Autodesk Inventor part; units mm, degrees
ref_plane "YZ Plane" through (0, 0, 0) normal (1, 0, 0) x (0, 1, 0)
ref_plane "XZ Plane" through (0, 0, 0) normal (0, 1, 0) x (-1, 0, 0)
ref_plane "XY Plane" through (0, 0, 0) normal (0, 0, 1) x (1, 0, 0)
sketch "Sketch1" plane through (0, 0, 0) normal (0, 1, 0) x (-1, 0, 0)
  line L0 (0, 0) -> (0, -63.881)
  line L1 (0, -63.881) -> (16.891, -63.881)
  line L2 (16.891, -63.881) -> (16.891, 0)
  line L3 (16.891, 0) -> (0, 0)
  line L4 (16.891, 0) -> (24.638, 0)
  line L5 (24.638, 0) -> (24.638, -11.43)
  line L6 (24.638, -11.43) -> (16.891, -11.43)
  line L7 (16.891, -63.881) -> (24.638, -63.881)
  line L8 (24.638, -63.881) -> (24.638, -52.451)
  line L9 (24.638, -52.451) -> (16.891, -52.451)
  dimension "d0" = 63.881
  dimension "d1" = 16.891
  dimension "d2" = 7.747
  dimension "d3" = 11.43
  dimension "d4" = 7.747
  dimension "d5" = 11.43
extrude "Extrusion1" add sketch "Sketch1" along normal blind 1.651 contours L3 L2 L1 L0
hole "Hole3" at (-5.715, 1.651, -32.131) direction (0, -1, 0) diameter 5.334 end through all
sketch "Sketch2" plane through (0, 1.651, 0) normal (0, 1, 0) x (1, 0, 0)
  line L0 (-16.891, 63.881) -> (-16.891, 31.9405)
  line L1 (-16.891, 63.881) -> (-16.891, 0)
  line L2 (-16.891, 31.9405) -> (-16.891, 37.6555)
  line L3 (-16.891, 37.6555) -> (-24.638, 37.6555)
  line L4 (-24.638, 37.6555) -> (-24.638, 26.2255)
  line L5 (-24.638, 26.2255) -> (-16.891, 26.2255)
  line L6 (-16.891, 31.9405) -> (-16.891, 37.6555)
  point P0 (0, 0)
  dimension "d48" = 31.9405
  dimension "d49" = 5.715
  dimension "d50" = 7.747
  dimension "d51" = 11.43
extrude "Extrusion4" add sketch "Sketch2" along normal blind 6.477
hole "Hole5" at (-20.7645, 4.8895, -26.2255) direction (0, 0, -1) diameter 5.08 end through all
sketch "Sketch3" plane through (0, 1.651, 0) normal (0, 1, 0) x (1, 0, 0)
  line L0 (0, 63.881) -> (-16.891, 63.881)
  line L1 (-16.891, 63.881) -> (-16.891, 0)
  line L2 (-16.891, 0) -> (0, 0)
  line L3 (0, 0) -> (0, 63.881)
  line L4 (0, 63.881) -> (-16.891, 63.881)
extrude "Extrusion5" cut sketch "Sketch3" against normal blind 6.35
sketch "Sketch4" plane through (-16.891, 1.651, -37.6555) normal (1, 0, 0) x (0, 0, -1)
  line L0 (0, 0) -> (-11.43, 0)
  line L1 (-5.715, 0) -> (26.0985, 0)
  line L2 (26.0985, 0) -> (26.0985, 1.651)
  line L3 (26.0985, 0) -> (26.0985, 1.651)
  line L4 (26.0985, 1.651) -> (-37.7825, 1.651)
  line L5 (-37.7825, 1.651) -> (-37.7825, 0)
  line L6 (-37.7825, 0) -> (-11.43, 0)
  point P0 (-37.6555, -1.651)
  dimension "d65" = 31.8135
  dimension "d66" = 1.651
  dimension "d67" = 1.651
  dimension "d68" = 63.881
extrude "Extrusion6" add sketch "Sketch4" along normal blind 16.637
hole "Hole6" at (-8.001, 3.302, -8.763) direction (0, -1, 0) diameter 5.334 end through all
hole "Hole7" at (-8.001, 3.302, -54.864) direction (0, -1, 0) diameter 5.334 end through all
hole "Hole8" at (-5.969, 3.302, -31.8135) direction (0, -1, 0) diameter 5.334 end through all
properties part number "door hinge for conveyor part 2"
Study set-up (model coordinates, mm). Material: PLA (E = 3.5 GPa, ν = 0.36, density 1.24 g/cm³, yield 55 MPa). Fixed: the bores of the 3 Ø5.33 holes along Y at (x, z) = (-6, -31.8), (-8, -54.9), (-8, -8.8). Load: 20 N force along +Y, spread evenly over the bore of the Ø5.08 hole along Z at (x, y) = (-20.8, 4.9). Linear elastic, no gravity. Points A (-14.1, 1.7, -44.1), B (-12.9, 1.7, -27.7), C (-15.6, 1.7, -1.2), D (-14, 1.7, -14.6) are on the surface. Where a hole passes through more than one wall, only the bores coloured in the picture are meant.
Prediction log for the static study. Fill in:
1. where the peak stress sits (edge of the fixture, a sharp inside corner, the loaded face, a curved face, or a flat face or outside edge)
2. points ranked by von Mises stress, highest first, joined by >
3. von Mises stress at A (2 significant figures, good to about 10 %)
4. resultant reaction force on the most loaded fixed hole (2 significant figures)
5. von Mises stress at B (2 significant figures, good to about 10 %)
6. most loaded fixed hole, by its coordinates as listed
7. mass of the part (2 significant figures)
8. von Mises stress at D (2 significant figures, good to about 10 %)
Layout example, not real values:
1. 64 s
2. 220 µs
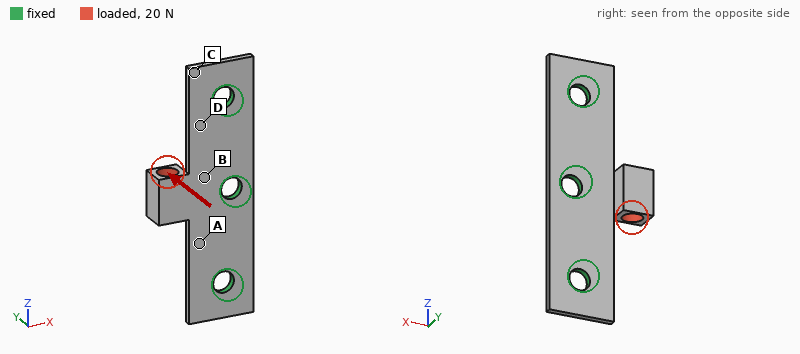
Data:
1. a flat face or outside edge
2. B > A > D > C
3. 8.4 MPa
4. 18 N
5. 14 MPa
6. (-6, -31.8)
7. 2.5 g
8. 5.2 MPa
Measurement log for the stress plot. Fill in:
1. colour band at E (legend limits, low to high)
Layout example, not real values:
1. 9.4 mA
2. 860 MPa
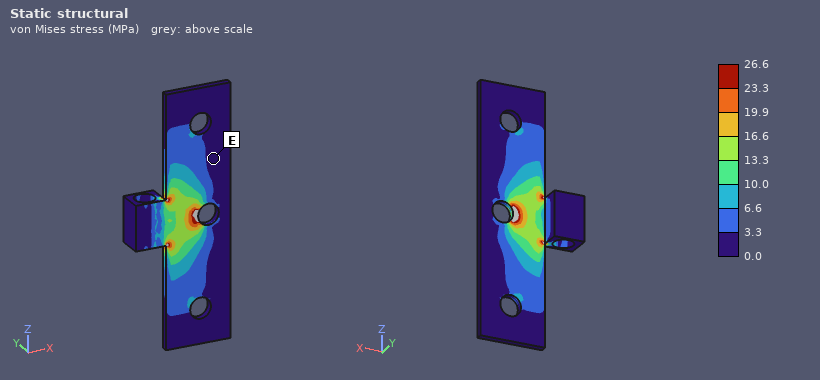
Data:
1. 0.0 to 3.3 MPa
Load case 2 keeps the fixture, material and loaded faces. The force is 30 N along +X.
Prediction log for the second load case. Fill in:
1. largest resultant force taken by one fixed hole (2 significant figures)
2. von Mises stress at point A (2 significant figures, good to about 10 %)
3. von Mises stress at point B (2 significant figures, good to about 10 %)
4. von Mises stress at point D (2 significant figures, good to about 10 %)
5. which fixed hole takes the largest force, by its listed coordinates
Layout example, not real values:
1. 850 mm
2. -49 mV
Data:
1. 26 N
2. 3.1 MPa
3. 5.7 MPa
4. 1.6 MPa
5. (-6, -31.8)
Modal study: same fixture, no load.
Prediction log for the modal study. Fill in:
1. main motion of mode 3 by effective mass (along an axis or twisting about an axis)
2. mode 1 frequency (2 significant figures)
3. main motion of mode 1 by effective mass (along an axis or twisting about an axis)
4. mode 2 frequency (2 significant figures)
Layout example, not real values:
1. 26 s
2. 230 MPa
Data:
1. along Y
2. 1300 Hz
3. along Y
4. 3700 Hz
